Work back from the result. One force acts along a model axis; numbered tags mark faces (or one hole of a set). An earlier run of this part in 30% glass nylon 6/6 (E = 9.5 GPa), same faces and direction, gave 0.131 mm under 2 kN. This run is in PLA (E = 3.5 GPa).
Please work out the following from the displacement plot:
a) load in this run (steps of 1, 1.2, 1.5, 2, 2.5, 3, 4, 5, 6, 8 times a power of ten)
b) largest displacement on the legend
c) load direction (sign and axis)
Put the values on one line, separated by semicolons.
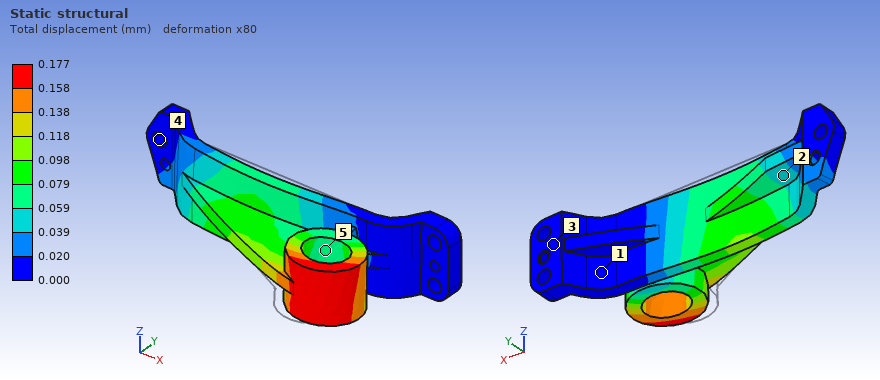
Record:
1 kN; 0.177 mm; +X
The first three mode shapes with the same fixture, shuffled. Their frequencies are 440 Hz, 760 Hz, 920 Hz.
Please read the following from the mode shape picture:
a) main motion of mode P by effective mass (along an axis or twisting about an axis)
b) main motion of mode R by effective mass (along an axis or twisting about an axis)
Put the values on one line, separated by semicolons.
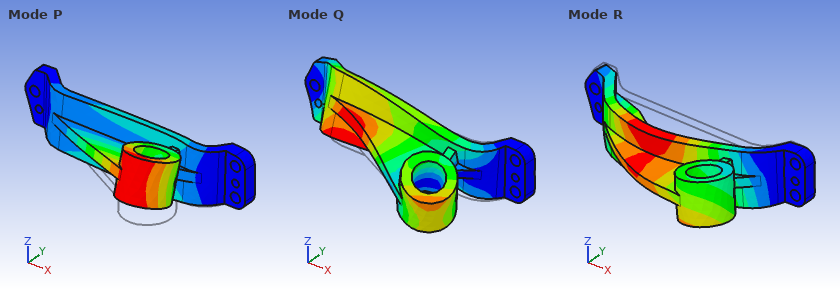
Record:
along Z; along Y
